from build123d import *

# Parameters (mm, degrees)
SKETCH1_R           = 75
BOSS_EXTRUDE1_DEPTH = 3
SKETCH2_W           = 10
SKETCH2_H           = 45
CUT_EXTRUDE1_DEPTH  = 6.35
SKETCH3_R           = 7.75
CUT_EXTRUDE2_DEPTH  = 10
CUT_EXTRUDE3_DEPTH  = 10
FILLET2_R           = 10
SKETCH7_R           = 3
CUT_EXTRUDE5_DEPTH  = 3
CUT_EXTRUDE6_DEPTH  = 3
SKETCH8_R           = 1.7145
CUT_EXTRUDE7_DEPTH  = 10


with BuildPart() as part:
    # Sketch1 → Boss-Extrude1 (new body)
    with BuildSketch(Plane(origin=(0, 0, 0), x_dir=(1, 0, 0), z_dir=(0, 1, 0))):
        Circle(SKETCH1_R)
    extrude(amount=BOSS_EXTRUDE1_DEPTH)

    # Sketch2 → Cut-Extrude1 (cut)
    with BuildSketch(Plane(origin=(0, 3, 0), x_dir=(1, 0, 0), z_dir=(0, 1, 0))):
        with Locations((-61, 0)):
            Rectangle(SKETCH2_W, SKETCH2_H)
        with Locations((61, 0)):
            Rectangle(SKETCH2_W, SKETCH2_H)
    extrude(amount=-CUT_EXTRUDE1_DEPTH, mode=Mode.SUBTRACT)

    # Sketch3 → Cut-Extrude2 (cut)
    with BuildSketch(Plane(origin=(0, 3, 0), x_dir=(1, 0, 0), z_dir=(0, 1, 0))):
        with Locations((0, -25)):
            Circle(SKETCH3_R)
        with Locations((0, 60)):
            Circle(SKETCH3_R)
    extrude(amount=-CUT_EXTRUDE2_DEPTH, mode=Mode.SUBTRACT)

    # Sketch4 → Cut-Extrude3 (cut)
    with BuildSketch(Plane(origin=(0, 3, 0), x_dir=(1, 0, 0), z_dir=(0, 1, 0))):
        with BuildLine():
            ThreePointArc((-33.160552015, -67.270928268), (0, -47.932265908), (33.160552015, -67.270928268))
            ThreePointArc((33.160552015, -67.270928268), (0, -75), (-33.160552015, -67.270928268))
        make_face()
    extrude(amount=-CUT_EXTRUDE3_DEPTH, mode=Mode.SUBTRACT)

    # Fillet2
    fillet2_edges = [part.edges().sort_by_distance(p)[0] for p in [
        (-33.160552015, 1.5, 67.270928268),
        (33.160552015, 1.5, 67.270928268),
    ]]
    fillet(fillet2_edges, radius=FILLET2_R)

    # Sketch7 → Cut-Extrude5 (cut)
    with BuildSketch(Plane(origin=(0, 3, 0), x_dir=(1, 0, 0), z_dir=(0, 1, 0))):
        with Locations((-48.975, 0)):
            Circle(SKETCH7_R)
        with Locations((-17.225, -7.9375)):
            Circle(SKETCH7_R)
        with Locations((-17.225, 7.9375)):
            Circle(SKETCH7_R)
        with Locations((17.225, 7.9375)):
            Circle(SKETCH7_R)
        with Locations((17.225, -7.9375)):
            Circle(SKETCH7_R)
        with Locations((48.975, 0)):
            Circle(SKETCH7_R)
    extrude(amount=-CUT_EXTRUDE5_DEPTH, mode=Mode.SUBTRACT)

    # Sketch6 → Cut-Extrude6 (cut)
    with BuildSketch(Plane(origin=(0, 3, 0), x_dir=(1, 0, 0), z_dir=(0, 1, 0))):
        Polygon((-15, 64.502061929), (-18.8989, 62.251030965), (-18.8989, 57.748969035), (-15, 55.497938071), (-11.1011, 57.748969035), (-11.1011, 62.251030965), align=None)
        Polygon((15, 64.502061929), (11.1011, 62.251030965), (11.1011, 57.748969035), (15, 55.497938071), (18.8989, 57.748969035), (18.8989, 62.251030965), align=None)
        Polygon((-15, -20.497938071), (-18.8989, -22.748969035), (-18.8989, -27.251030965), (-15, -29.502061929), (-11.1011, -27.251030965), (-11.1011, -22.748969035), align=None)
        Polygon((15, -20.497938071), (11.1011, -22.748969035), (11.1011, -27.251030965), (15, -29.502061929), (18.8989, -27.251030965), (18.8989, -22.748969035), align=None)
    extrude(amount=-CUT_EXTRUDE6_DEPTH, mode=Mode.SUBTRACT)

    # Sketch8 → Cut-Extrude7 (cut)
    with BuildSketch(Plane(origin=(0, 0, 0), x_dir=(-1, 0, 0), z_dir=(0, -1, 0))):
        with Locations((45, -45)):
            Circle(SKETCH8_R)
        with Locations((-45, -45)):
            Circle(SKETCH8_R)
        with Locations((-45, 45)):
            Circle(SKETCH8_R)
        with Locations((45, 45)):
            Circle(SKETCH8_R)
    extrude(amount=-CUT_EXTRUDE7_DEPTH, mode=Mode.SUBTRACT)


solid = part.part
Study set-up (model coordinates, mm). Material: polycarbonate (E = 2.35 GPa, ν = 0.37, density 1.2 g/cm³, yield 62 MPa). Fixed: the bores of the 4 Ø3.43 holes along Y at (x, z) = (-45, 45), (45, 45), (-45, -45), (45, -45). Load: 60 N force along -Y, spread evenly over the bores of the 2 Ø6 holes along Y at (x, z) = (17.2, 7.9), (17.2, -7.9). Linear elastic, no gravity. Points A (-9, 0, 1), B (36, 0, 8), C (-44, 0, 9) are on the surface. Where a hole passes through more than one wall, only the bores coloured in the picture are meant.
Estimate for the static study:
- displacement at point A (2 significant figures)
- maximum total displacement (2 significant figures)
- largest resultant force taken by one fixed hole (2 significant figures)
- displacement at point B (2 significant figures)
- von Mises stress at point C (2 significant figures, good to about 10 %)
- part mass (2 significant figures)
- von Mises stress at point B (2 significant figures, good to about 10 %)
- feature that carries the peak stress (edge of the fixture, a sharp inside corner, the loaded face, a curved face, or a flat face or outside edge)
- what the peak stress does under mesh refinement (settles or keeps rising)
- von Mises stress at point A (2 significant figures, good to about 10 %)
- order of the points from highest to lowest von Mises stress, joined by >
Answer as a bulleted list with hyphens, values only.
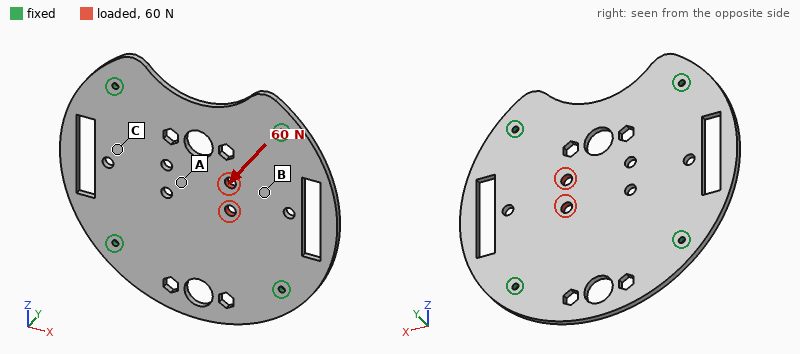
- 0.86 mm
- 1.2 mm
- 22 N
- 0.77 mm
- 1.3 MPa
- 53 g
- 4.2 MPa
- edge of the fixture
- keeps rising
- 3.0 MPa
- B > A > C
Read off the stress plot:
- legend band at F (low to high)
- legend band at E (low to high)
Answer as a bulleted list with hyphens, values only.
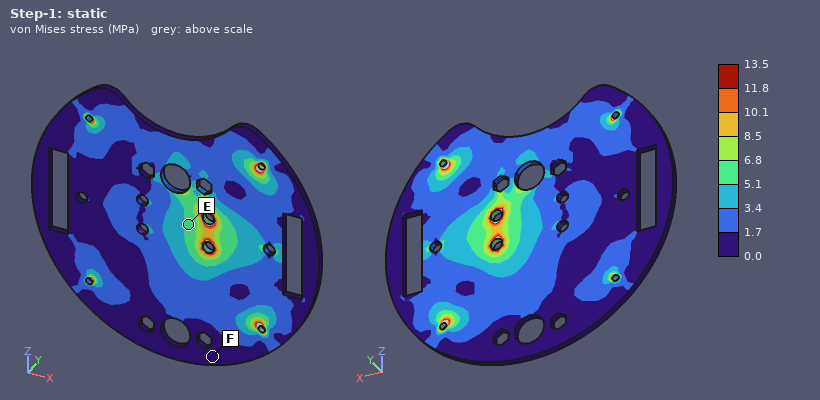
- 0.0 to 1.7 MPa
- 5.1 to 6.8 MPa
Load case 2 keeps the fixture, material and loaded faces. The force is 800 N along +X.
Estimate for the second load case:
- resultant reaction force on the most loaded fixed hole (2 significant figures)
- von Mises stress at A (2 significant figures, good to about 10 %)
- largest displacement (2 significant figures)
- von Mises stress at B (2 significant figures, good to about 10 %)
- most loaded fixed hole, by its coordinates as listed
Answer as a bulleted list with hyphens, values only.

- 260 N
- 2.6 MPa
- 0.13 mm
- 2.2 MPa
- (45, -45)
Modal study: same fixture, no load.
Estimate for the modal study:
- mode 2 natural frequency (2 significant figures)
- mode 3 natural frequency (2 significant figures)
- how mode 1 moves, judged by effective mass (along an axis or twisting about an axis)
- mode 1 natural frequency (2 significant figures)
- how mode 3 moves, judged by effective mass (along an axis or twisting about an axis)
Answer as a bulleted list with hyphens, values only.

- 420 Hz
- 460 Hz
- along Y
- 350 Hz
- twisting about Z
